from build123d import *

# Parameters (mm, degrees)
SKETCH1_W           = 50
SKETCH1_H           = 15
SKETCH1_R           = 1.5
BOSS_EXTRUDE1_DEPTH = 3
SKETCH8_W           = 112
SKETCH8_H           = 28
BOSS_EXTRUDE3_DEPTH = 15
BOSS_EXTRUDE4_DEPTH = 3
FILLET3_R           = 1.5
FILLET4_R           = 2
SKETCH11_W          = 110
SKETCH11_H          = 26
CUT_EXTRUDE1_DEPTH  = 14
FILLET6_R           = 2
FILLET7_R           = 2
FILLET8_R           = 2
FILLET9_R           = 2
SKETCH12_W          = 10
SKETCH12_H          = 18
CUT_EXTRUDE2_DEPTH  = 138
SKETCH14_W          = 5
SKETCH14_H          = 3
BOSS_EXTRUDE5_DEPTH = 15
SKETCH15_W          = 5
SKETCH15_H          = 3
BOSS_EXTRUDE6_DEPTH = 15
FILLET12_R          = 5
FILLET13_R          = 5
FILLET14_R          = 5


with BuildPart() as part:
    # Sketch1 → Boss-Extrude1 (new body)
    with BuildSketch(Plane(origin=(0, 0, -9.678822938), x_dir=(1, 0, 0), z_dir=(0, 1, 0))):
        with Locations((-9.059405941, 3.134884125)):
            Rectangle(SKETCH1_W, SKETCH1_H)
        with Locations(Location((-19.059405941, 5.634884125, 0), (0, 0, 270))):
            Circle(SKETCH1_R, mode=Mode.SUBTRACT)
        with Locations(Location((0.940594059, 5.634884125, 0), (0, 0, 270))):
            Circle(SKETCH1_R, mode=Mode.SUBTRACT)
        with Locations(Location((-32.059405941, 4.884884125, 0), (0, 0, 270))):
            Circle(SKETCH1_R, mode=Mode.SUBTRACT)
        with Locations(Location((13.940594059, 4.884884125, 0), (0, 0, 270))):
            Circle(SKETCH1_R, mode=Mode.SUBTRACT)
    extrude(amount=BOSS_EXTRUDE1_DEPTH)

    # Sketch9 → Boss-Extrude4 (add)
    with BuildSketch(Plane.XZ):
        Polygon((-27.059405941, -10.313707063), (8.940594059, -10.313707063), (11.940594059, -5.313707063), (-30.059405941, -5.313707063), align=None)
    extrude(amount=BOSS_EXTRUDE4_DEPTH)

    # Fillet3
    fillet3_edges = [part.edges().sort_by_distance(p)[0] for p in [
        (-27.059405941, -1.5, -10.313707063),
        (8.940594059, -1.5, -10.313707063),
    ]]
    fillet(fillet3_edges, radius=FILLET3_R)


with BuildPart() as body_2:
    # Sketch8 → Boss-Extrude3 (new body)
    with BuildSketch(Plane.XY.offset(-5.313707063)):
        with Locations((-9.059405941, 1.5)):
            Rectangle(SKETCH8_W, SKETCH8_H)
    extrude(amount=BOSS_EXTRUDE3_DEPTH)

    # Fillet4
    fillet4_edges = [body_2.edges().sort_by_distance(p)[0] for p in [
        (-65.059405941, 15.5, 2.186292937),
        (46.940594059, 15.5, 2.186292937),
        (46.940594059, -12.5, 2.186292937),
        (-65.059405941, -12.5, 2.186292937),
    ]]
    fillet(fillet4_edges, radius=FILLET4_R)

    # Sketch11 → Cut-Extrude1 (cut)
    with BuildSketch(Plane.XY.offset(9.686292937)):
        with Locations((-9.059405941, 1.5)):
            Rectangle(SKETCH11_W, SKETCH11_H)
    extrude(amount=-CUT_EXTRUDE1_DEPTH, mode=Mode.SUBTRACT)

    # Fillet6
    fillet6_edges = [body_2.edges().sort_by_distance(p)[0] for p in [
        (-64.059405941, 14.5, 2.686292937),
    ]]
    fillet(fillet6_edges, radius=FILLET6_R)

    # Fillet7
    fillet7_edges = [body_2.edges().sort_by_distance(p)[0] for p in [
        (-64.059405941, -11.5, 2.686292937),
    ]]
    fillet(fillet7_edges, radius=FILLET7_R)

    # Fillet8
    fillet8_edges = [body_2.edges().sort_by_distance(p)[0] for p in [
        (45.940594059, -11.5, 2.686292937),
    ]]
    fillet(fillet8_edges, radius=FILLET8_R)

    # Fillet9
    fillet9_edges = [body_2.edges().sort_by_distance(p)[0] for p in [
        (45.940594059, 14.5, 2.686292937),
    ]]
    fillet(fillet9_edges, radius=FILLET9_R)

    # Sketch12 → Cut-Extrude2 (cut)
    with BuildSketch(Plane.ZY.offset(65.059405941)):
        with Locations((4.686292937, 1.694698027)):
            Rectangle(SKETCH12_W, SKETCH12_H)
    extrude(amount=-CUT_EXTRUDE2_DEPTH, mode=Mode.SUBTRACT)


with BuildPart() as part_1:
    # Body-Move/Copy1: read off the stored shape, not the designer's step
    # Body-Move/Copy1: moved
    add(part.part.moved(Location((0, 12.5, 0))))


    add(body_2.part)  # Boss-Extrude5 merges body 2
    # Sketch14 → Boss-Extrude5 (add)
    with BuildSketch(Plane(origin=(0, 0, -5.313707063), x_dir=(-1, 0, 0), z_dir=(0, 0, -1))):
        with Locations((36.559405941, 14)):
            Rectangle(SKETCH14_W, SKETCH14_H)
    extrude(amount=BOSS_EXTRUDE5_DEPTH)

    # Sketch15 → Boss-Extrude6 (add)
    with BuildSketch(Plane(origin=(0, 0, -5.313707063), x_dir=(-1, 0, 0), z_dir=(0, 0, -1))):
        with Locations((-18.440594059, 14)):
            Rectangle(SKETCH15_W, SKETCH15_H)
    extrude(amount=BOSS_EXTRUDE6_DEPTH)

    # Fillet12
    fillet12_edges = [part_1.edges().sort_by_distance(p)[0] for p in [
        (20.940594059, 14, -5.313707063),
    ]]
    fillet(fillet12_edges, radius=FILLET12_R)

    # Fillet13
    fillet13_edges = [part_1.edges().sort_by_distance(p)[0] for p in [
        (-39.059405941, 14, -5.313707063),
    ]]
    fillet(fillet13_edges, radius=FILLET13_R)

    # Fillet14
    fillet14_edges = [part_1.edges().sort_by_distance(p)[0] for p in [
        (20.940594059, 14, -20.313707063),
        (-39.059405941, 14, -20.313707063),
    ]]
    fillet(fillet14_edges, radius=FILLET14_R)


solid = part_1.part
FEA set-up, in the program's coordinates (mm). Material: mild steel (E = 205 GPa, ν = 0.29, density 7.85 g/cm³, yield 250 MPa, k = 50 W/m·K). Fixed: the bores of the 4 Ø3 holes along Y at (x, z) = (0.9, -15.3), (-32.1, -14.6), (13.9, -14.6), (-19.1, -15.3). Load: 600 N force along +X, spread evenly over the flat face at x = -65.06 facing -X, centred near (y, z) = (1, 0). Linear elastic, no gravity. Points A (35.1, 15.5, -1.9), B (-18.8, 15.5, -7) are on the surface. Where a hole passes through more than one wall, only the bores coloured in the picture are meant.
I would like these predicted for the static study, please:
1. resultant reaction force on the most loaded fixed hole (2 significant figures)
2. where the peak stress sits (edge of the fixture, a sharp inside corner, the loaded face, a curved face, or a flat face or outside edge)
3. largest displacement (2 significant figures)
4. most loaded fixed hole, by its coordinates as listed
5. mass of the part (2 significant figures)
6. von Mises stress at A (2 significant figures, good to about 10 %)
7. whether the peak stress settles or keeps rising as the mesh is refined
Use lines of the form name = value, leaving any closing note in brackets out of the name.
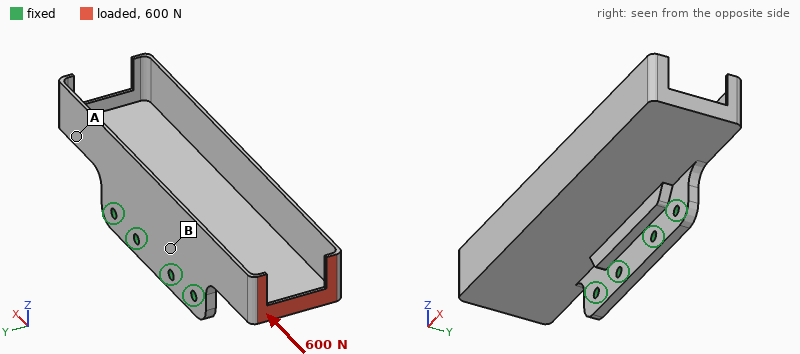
resultant reaction force on the most loaded fixed hole = 290 N
where the peak stress sits = a sharp inside corner
largest displacement = 0.15 mm
most loaded fixed hole, by its coordinates as listed = (-32.1, -14.6)
mass of the part = 77 g
von Mises stress at A = 25 MPa
whether the peak stress settles or keeps rising as the mesh is refined = keeps rising
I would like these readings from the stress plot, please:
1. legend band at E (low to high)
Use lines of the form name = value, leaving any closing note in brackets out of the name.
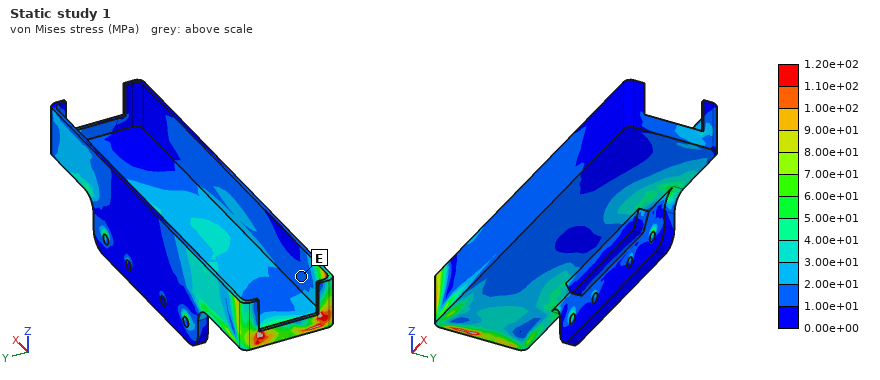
legend band at E = 1.00e+01 to 2.00e+01 MPa
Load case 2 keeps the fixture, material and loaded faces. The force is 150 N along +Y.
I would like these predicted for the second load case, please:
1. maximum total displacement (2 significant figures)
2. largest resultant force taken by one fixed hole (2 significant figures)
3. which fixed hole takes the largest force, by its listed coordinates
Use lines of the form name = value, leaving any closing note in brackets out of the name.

maximum total displacement = 0.30 mm
largest resultant force taken by one fixed hole = 230 N
which fixed hole takes the largest force, by its listed coordinates = (-32.1, -14.6)
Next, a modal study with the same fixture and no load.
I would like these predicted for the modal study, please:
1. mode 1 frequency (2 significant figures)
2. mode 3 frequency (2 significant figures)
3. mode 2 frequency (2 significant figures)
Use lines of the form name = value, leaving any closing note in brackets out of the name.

mode 1 frequency = 680 Hz
mode 3 frequency = 2900 Hz
mode 2 frequency = 680 Hz
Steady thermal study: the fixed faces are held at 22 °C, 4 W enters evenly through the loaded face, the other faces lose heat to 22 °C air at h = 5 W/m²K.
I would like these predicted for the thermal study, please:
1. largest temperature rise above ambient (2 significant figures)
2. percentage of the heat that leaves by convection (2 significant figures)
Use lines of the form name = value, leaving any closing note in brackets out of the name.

largest temperature rise above ambient = 60 K
percentage of the heat that leaves by convection = 23 %
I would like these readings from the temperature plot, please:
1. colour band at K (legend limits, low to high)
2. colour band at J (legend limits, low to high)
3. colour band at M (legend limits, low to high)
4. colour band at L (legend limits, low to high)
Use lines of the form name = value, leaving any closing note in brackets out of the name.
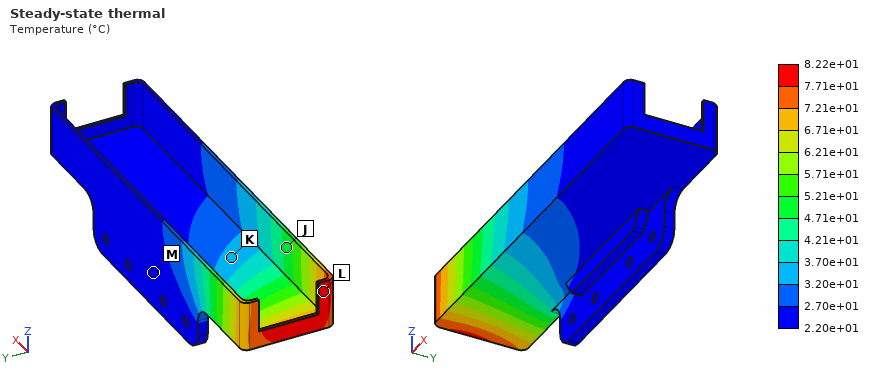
colour band at K = 3.20e+01 to 3.70e+01 °C
colour band at J = 4.71e+01 to 5.21e+01 °C
colour band at M = 2.20e+01 to 2.70e+01 °C
colour band at L = 7.71e+01 to 8.22e+01 °C
